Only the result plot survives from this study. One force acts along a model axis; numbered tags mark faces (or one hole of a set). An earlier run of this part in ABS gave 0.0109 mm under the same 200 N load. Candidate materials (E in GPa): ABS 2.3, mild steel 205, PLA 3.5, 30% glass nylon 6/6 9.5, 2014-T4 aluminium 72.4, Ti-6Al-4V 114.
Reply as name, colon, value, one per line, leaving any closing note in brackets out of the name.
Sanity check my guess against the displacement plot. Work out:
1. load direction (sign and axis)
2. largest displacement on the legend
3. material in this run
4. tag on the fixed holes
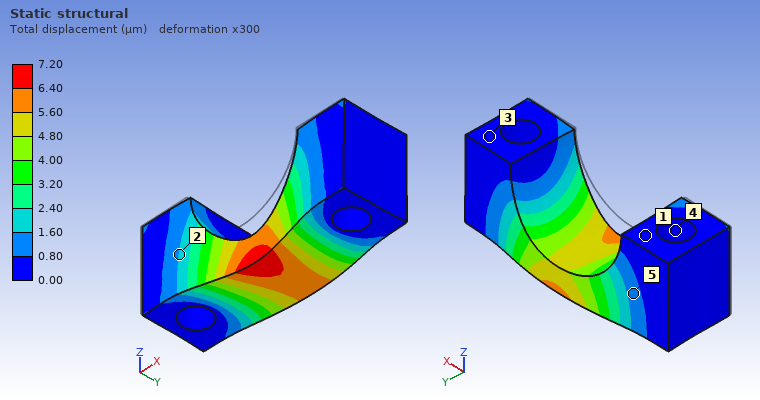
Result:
load direction: +Y
largest displacement on the legend: 7.20 µm
material in this run: PLA
tag on the fixed holes: 4
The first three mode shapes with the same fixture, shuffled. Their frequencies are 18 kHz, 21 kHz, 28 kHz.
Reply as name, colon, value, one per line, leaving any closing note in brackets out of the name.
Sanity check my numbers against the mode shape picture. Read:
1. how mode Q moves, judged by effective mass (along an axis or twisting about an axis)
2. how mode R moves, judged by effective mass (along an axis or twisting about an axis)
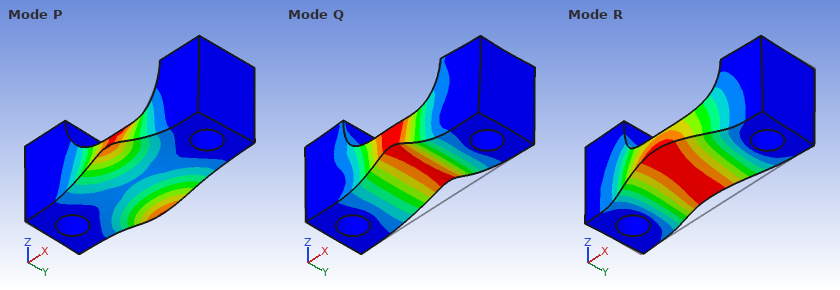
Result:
how mode Q moves, judged by effective mass: along Z
how mode R moves, judged by effective mass: along Y
